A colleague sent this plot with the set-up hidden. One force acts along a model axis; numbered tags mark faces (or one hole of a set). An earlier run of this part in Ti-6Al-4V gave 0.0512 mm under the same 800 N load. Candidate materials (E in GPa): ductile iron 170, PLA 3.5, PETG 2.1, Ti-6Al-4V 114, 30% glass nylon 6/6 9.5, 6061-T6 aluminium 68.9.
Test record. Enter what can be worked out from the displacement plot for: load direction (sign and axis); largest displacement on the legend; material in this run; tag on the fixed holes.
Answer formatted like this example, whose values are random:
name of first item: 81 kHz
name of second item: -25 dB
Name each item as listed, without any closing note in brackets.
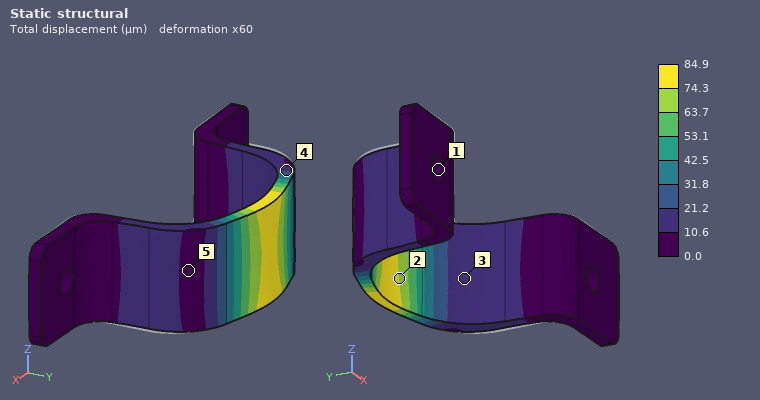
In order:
load direction: +Y
largest displacement on the legend: 84.9 µm
material in this run: 6061-T6 aluminium
tag on the fixed holes: 1
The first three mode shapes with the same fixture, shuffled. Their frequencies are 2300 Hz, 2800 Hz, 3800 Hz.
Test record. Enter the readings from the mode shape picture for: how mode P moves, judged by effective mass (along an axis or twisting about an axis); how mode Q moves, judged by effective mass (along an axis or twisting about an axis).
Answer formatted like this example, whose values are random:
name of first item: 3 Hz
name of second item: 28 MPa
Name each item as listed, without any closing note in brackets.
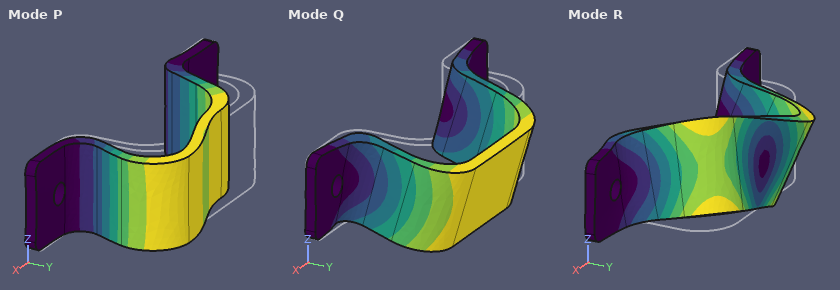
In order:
how mode P moves, judged by effective mass: along X
how mode Q moves, judged by effective mass: along Z
